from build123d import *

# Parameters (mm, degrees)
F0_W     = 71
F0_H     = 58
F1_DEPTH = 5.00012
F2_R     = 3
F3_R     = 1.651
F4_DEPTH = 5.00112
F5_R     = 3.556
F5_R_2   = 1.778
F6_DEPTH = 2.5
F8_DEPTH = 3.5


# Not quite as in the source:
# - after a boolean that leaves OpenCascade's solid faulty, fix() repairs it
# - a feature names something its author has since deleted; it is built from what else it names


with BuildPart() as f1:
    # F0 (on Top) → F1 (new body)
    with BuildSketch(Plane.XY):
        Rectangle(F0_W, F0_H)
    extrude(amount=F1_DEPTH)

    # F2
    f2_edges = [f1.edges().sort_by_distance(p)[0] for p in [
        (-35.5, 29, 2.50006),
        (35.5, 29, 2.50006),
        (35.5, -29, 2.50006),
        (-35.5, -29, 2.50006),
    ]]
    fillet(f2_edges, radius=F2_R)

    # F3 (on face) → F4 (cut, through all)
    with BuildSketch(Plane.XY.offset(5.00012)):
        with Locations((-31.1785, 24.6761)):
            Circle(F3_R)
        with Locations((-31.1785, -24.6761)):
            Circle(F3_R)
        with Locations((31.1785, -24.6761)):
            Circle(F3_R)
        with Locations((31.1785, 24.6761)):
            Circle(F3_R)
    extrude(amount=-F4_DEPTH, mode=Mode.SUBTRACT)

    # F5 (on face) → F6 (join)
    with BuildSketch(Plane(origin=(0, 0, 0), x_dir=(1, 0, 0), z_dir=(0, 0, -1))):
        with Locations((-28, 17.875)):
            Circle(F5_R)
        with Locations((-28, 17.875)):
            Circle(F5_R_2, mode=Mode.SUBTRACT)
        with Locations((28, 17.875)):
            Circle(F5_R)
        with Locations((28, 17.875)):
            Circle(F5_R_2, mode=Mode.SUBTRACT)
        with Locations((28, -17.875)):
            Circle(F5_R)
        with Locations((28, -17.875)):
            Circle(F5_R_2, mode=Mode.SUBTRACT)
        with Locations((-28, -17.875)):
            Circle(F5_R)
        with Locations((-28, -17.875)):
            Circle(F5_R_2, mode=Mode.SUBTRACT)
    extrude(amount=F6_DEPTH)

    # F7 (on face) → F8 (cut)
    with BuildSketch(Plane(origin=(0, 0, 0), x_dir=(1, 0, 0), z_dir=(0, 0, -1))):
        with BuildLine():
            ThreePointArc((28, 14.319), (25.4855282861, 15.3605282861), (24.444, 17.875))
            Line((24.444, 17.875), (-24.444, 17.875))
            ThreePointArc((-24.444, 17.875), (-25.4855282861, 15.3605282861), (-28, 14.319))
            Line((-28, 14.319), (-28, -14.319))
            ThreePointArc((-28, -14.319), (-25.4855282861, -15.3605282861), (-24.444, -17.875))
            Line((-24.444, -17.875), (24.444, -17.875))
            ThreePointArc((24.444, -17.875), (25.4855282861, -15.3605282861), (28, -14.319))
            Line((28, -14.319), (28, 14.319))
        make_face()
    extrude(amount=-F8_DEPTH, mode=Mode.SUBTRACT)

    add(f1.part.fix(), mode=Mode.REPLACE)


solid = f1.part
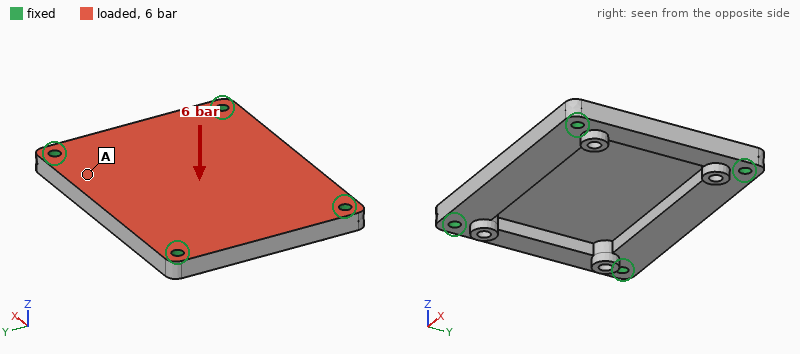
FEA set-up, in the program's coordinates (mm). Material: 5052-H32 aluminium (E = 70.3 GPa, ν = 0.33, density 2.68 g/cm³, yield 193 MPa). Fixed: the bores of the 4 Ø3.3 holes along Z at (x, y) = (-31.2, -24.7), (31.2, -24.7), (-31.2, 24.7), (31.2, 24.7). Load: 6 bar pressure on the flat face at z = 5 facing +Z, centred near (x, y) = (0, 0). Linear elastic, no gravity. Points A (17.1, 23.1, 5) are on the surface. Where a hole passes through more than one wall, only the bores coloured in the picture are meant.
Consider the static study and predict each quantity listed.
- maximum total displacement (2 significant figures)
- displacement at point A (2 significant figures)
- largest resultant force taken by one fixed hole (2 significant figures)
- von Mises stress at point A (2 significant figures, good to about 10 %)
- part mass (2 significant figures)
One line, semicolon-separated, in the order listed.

0.23 mm; 0.038 mm; 780 N; 21 MPa; 37 g
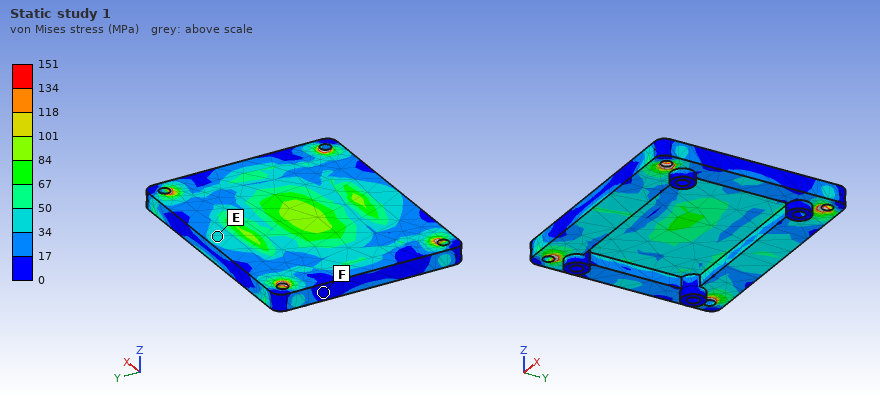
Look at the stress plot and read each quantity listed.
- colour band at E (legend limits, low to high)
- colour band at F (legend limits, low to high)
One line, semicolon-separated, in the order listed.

34 to 50 MPa; 0 to 17 MPa
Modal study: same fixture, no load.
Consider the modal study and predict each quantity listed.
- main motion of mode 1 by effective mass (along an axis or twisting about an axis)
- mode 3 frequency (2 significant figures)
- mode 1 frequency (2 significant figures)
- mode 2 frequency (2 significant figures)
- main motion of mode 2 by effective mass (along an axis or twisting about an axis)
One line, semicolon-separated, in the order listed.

along Z; 8100 Hz; 4900 Hz; 6500 Hz; twisting about X
